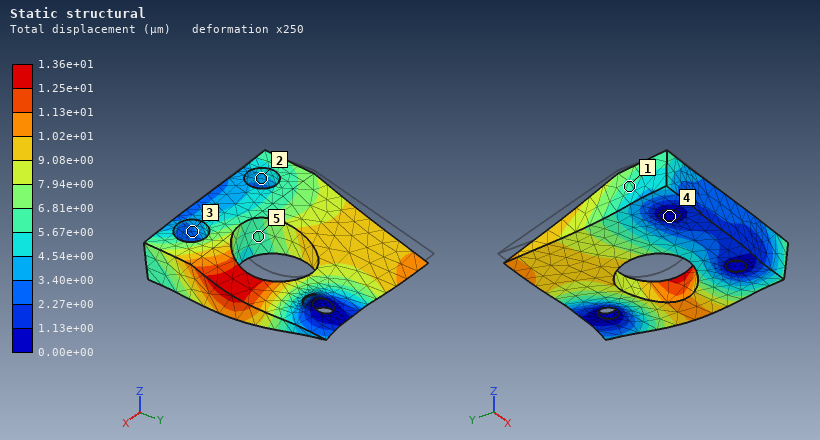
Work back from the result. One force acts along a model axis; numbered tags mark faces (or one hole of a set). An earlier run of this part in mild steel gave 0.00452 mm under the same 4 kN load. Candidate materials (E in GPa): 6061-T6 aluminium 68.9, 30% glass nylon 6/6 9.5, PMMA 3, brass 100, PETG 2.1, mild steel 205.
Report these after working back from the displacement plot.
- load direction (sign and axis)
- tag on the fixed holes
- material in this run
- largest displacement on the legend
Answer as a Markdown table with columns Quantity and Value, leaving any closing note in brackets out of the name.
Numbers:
| Quantity | Value |
|---|---|
| load direction | +X |
| tag on the fixed holes | 4 |
| material in this run | 6061-T6 aluminium |
| largest displacement on the legend | 1.36e+01 µm |
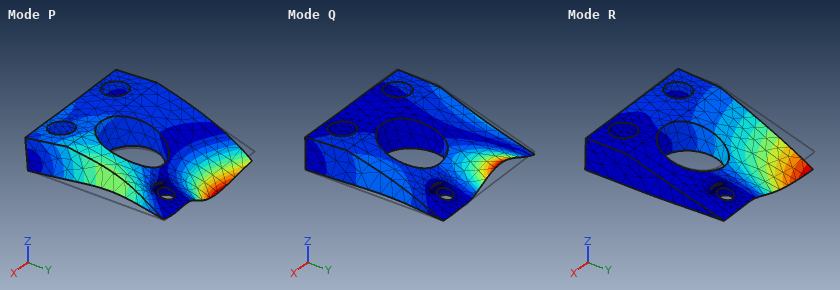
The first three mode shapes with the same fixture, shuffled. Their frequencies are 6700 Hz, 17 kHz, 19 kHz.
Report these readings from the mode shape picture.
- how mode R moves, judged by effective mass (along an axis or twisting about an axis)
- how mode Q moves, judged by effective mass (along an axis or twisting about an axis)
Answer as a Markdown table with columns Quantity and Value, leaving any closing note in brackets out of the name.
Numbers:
| Quantity | Value |
|---|---|
| how mode R moves, judged by effective mass | along Z |
| how mode Q moves, judged by effective mass | twisting about Y |
